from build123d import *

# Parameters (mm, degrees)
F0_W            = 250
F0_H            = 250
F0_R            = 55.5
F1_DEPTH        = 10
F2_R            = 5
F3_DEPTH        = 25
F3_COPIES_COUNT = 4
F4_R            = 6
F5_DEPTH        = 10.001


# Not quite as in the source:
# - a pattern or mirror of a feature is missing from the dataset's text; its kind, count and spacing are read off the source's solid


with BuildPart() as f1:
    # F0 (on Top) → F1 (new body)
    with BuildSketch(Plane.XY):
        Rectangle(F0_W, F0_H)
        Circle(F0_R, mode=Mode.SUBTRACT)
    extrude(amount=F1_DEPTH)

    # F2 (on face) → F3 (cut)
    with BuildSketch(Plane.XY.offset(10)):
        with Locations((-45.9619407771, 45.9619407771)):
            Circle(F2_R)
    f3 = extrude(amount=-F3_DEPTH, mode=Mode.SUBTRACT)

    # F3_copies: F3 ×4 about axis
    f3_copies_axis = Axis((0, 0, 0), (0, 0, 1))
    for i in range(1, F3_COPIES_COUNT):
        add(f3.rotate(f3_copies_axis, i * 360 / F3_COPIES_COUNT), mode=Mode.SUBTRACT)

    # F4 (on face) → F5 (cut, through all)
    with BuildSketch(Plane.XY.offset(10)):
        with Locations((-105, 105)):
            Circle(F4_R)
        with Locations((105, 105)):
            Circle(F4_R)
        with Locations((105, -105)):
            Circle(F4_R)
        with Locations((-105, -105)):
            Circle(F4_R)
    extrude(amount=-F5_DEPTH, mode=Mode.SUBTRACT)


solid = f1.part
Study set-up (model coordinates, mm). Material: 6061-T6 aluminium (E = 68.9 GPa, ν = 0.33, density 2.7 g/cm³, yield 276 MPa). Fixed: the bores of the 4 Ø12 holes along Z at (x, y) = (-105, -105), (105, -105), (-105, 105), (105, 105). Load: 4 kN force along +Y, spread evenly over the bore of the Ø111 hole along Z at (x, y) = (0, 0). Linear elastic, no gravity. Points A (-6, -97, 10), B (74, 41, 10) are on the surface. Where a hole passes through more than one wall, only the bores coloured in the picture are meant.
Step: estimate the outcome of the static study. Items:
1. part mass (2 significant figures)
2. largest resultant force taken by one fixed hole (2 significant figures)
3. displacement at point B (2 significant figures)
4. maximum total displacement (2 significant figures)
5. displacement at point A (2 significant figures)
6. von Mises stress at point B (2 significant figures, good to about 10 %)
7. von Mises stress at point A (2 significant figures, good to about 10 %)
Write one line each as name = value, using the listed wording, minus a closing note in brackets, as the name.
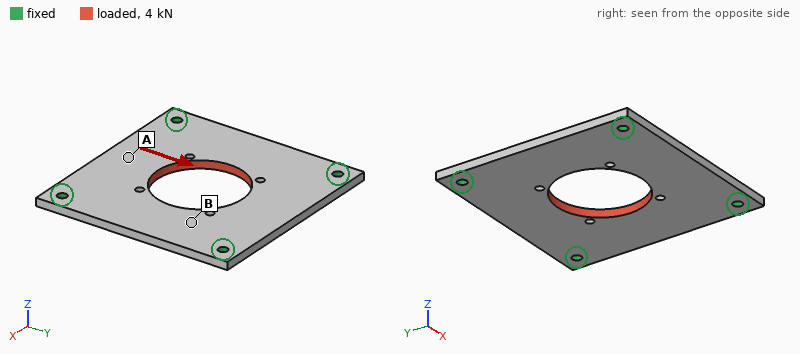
part mass = 1.4 kg
largest resultant force taken by one fixed hole = 1.1 kN
displacement at point B = 2.3 µm
maximum total displacement = 4.7 µm
displacement at point A = 4.3 µm
von Mises stress at point B = 1.5 MPa
von Mises stress at point A = 0.67 MPa
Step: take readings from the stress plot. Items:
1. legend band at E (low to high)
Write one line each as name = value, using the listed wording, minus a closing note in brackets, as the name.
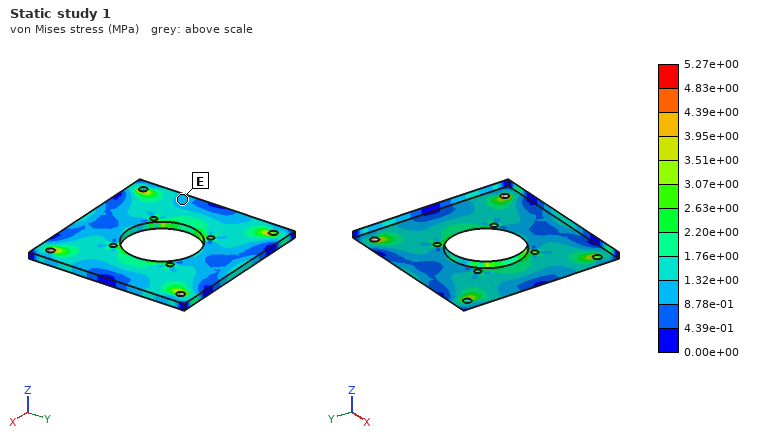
legend band at E = 8.78e-01 to 1.32e+00 MPa
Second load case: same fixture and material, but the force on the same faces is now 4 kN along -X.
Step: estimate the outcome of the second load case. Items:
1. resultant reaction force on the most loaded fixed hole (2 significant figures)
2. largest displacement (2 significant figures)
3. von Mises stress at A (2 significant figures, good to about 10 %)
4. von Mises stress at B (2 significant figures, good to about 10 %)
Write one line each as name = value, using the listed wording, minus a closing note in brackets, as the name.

resultant reaction force on the most loaded fixed hole = 1.1 kN
largest displacement = 4.7 µm
von Mises stress at A = 1.2 MPa
von Mises stress at B = 1.5 MPa
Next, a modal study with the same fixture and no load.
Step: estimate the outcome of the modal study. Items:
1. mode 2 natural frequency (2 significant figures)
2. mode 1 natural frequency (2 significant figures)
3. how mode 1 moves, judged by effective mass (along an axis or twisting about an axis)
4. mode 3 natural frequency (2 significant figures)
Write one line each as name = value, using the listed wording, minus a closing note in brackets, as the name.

mode 2 natural frequency = 1200 Hz
mode 1 natural frequency = 880 Hz
how mode 1 moves, judged by effective mass = along Z
mode 3 natural frequency = 1200 Hz
